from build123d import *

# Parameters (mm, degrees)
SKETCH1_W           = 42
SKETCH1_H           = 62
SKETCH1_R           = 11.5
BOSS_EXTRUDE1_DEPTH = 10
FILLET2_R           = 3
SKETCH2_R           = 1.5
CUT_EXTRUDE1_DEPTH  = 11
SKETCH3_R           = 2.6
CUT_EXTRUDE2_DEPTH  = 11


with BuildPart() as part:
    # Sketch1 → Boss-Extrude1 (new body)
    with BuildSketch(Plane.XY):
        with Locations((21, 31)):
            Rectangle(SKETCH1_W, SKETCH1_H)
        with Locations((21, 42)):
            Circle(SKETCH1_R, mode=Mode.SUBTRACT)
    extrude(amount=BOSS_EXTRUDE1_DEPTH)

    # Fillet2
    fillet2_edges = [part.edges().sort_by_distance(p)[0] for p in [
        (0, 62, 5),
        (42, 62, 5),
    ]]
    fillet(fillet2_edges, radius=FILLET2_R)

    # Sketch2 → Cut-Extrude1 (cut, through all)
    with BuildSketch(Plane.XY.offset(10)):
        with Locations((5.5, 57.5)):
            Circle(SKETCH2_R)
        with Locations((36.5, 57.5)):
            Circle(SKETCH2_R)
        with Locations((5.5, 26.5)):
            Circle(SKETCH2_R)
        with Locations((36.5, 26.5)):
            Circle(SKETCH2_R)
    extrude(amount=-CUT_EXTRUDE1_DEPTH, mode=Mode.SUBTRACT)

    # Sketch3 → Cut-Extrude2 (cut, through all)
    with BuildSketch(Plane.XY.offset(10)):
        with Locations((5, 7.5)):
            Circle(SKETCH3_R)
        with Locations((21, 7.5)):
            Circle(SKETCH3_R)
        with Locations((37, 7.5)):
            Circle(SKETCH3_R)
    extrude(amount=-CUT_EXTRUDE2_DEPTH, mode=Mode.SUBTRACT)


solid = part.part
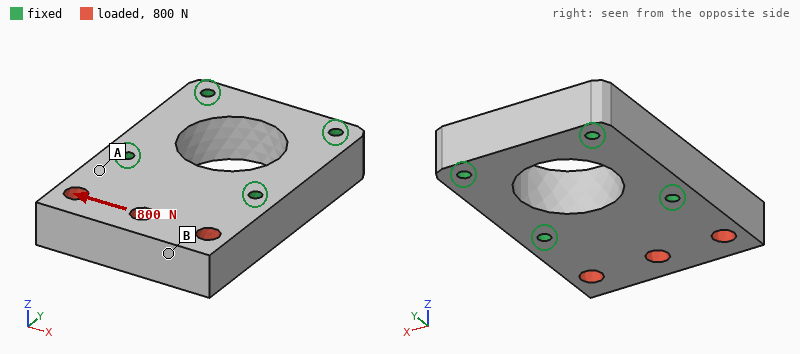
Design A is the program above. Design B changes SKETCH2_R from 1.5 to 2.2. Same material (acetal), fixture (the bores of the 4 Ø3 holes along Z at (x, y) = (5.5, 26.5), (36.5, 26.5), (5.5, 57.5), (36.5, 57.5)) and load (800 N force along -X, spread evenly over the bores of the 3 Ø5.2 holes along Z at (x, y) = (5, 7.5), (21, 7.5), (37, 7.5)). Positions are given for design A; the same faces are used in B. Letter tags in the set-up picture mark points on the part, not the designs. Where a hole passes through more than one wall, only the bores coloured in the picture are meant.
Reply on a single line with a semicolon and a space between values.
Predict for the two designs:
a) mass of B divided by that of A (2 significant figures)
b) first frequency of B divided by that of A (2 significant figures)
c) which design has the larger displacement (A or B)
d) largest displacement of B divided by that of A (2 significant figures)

0.98; 1.1; A; 0.92
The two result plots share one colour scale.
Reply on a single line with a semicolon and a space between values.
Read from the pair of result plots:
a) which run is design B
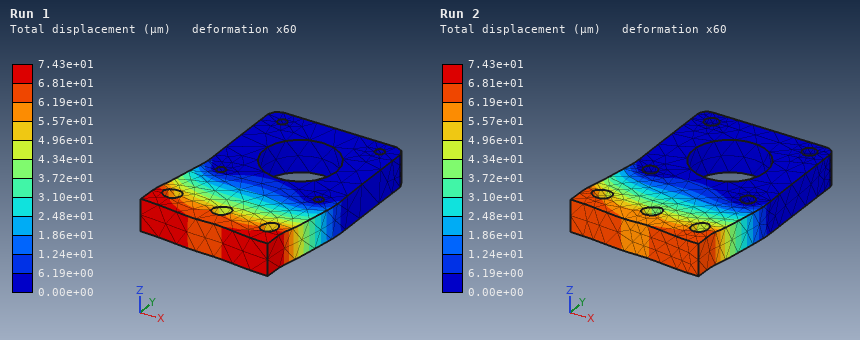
Run 2
